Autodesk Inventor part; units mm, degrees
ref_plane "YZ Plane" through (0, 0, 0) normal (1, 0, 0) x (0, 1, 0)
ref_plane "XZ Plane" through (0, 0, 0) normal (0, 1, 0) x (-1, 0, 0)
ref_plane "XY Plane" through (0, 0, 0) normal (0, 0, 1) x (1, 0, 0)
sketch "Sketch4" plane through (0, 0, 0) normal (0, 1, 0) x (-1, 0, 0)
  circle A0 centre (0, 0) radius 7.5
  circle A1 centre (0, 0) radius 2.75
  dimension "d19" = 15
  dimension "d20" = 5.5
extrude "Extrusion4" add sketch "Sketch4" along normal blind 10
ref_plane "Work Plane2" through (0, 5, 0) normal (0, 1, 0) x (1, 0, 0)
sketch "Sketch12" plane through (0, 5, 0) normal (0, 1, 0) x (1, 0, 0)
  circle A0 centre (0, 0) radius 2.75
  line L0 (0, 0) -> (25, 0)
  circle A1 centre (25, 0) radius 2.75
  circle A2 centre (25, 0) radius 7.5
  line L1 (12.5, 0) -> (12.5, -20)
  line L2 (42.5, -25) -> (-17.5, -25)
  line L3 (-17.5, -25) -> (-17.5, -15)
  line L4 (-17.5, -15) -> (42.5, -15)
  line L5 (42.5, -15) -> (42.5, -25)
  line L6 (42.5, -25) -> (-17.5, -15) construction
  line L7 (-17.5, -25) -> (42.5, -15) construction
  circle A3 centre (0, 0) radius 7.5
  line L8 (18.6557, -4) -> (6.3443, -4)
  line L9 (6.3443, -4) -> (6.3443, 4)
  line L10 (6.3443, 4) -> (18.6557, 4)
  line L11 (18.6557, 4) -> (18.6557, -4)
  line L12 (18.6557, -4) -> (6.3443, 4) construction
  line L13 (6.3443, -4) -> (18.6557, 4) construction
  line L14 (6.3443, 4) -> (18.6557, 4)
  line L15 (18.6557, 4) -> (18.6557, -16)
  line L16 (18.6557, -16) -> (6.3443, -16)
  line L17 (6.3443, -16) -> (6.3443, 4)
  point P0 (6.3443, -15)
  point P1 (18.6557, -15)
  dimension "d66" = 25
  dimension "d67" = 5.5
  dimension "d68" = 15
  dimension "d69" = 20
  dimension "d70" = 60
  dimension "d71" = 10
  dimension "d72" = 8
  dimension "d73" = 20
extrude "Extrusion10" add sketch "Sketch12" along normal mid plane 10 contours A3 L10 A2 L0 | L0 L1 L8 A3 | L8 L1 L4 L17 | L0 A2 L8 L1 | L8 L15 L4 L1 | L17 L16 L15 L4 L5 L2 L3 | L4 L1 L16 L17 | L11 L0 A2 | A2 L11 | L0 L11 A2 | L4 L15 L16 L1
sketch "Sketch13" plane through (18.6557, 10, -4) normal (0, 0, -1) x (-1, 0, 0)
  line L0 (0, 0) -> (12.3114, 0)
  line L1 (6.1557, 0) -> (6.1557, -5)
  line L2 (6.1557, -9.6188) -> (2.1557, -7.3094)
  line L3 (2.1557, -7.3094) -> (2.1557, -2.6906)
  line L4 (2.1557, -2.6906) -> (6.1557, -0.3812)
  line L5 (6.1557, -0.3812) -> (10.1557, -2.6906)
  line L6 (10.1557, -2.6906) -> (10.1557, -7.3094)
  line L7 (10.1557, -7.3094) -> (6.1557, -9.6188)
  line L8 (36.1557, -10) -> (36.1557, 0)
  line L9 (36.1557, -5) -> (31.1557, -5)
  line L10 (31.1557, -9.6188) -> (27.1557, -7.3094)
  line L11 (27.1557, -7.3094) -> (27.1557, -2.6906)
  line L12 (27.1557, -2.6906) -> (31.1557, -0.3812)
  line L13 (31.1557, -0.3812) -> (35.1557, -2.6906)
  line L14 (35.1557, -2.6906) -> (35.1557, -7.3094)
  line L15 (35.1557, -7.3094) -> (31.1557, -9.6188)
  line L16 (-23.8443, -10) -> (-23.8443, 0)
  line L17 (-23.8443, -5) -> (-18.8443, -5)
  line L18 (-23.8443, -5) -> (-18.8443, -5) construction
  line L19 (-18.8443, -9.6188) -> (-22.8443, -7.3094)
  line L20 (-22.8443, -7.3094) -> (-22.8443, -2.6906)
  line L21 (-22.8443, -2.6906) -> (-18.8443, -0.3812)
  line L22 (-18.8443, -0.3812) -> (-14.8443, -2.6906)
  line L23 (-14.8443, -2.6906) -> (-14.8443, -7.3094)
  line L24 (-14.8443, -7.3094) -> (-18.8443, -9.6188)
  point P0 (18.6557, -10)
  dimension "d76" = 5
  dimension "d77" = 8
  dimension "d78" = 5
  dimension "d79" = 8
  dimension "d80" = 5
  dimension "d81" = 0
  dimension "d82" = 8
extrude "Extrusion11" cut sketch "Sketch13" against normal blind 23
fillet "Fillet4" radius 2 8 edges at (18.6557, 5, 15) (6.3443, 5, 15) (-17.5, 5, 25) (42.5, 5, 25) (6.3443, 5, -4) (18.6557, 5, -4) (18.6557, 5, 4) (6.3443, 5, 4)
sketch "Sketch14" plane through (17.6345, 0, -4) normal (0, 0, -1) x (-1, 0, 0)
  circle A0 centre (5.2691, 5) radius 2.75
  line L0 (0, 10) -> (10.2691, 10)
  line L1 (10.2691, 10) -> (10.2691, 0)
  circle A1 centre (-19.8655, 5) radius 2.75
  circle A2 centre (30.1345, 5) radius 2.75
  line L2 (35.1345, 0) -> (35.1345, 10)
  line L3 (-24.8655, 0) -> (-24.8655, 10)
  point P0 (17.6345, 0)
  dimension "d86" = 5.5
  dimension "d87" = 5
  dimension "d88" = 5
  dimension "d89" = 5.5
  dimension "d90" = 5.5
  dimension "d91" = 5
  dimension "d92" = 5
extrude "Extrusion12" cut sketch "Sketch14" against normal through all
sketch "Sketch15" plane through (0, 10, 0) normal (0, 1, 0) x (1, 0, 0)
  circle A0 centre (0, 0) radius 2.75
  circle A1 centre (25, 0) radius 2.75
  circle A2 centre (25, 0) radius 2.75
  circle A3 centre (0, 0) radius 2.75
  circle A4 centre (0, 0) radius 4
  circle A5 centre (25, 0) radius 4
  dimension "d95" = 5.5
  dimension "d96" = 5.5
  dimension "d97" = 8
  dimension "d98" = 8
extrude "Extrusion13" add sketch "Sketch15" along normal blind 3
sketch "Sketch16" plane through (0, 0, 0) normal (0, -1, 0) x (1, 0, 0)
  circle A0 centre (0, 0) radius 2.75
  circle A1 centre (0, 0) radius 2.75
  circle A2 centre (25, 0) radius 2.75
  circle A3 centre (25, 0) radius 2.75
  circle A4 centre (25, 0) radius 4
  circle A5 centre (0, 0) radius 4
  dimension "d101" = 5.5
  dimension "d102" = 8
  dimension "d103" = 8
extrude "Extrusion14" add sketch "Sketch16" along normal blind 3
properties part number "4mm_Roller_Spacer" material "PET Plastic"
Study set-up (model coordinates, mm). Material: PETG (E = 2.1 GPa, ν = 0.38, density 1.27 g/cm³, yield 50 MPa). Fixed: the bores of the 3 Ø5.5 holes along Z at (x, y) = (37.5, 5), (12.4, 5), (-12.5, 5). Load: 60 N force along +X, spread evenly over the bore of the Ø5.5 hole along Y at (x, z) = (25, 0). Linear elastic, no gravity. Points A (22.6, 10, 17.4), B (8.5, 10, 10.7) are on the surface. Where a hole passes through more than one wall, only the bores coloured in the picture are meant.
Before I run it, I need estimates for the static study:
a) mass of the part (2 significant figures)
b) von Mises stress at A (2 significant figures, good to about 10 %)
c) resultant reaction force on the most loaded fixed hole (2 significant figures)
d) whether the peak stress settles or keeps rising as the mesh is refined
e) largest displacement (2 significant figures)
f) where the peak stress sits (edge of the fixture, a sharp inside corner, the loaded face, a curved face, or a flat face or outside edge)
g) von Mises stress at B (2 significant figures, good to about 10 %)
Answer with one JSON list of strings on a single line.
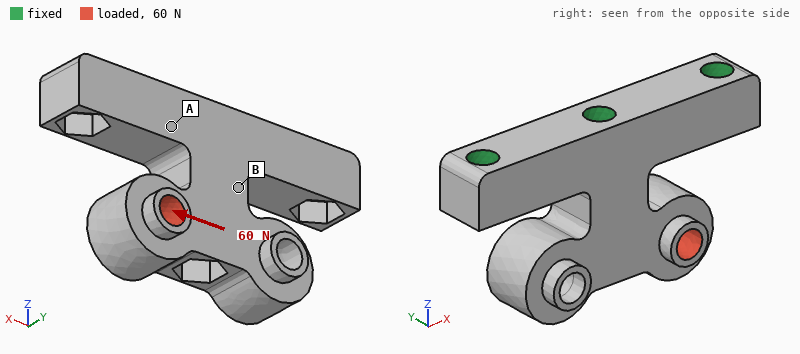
["12 g", "1.1 MPa", "35 N", "keeps rising", "0.16 mm", "a sharp inside corner", "2.7 MPa"]
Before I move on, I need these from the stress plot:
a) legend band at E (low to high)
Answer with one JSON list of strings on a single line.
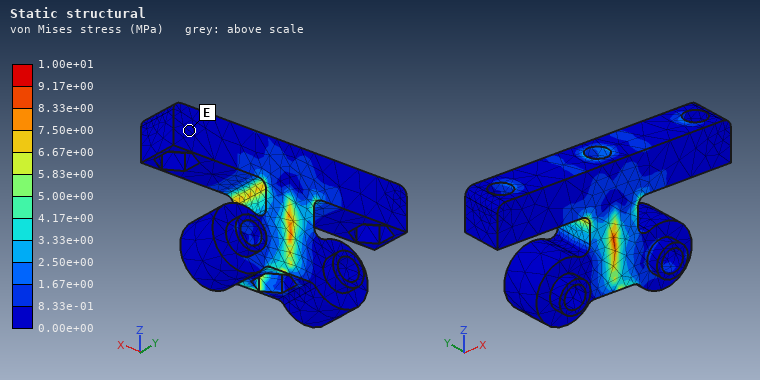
["0.00e+00 to 8.33e-01 MPa"]
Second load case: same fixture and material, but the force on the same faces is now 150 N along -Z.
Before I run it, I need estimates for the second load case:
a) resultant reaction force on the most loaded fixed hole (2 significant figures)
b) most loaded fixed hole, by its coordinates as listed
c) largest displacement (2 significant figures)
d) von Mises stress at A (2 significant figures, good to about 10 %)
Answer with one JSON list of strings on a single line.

["150 N", "(12.4, 5)", "0.45 mm", "1.8 MPa"]
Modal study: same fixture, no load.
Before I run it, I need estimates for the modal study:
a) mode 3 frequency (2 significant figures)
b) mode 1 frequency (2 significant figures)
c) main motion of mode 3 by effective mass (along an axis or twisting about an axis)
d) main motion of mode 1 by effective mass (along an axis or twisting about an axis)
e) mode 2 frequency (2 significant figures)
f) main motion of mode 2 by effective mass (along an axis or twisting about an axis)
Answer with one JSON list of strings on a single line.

["1500 Hz", "1300 Hz", "twisting about Z", "along Y", "1400 Hz", "along X"]
